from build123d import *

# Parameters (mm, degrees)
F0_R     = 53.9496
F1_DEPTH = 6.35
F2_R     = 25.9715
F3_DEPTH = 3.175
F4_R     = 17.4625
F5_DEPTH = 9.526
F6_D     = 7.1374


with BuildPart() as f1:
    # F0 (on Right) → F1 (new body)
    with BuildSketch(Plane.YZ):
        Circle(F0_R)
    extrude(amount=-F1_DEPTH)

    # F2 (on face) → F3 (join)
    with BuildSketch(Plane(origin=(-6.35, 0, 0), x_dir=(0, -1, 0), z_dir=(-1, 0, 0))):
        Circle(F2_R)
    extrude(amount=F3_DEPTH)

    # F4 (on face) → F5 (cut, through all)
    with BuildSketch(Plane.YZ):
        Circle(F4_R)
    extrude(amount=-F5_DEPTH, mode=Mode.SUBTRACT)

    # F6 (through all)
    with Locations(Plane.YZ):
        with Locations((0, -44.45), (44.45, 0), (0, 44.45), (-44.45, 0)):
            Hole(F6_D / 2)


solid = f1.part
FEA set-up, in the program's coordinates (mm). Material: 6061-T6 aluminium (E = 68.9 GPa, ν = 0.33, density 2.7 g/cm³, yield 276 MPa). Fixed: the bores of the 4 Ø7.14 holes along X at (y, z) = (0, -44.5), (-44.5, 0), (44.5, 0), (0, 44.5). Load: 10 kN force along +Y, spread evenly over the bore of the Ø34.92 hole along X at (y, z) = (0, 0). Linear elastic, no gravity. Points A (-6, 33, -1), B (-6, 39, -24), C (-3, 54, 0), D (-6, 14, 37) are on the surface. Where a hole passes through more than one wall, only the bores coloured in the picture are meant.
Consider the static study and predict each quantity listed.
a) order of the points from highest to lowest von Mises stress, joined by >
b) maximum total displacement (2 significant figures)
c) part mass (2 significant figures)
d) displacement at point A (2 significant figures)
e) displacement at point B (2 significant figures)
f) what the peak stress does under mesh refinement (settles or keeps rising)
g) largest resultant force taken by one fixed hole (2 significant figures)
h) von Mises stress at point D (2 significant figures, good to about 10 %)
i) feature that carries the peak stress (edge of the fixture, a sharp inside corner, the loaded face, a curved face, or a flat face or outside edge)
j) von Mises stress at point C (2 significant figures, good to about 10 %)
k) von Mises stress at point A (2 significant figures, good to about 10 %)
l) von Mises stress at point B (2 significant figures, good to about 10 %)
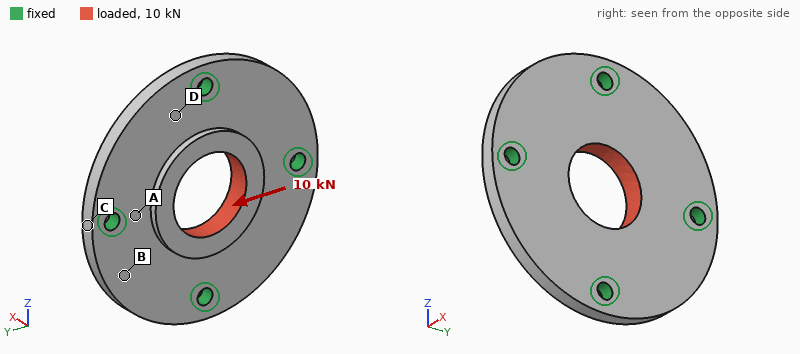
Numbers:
A > C > D > B
10 µm
150 g
3.3 µm
5.7 µm
keeps rising
3.0 kN
8.3 MPa
edge of the fixture
14 MPa
30 MPa
4.1 MPa
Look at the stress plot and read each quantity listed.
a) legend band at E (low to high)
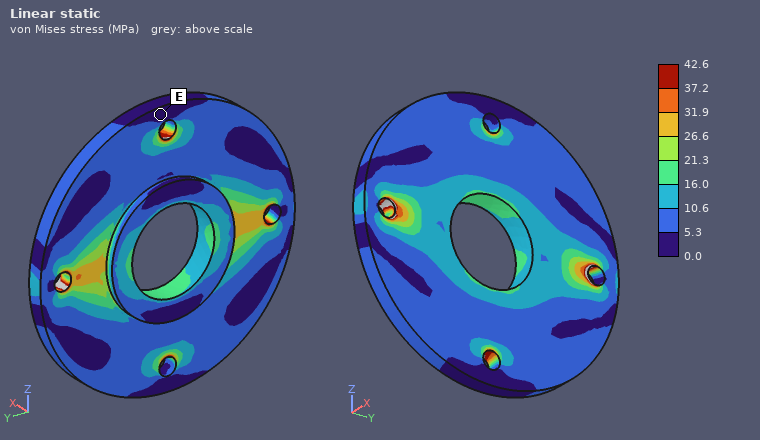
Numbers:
0.0 to 5.3 MPa
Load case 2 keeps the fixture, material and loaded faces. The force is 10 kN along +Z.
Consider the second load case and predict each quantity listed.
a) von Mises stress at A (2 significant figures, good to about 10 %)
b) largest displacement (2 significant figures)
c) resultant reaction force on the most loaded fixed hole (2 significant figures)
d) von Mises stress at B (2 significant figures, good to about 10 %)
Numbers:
7.2 MPa
10 µm
3.0 kN
5.8 MPa
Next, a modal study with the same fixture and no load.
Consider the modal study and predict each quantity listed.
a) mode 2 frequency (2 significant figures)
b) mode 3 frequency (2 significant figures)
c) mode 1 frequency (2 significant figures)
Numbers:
6900 Hz
6900 Hz
6600 Hz
